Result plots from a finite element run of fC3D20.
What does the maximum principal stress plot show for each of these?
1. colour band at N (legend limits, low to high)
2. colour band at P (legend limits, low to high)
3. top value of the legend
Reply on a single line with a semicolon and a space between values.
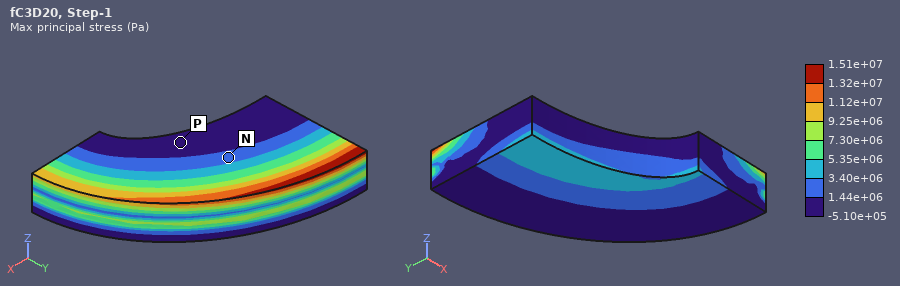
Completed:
1.44e+06 to 3.40e+06 Pa; -5.10e+05 to 1.44e+06 Pa; 1.51e+07 Pa
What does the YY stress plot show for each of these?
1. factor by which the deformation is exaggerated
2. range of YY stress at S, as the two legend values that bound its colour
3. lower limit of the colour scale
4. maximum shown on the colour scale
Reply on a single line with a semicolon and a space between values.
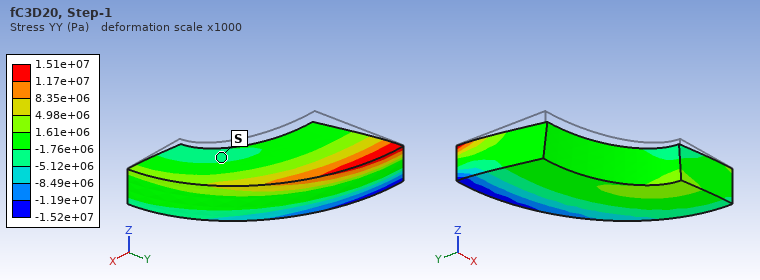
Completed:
1000; -5.12e+06 to -1.76e+06 Pa; -1.52e+07 Pa; 1.51e+07 Pa
